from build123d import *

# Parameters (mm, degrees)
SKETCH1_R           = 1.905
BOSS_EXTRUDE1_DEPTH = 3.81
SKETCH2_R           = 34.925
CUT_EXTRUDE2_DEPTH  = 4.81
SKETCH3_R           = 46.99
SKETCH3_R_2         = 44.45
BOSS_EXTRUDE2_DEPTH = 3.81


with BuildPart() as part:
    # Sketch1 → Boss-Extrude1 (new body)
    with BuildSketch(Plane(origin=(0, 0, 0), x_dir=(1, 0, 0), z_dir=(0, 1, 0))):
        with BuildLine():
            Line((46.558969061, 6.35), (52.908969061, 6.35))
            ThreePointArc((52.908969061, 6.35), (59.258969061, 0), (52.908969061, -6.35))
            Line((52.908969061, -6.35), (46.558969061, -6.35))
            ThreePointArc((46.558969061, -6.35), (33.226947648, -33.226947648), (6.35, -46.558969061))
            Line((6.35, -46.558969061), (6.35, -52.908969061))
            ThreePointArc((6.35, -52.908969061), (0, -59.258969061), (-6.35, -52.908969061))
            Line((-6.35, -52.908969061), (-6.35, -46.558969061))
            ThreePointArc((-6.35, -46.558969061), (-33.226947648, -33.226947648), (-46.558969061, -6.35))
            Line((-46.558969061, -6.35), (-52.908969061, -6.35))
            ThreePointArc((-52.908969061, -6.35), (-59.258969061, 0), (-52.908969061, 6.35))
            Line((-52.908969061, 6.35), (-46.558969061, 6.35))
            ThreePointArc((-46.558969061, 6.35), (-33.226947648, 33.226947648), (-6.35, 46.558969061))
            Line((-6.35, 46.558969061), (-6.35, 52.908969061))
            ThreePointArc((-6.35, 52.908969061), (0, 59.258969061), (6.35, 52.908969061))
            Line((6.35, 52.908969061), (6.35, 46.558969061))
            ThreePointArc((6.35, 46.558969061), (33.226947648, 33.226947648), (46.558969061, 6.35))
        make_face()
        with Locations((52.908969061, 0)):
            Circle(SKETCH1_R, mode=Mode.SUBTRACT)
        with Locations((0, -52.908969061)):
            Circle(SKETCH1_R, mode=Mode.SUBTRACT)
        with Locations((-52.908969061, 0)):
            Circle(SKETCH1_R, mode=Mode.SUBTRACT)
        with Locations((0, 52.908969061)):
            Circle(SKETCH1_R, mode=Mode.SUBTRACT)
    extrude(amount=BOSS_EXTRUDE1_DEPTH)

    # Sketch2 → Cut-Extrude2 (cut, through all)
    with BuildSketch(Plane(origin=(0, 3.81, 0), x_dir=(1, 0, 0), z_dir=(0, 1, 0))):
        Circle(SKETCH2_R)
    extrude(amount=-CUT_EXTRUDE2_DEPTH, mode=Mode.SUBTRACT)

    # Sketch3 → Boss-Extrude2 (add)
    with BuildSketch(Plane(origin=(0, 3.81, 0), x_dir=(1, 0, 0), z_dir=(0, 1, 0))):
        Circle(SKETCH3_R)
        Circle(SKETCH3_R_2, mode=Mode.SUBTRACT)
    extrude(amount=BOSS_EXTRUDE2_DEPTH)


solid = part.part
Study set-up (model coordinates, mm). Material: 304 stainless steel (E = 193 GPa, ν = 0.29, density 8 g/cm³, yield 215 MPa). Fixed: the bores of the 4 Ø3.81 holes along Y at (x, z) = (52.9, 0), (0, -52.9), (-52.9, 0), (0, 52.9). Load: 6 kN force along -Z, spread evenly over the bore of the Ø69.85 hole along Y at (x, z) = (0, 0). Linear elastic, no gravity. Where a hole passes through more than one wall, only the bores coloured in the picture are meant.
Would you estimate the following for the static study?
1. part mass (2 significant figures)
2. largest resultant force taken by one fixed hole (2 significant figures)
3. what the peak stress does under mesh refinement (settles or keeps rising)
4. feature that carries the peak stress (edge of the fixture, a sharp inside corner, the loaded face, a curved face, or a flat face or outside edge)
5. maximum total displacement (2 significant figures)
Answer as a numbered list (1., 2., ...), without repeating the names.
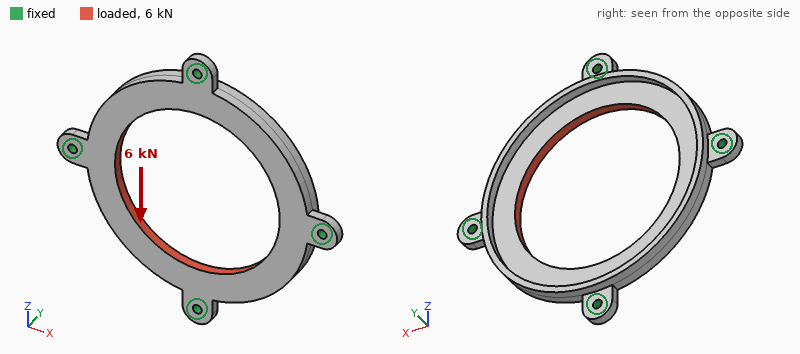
1. 130 g
2. 1.7 kN
3. keeps rising
4. edge of the fixture
5. 16 µm
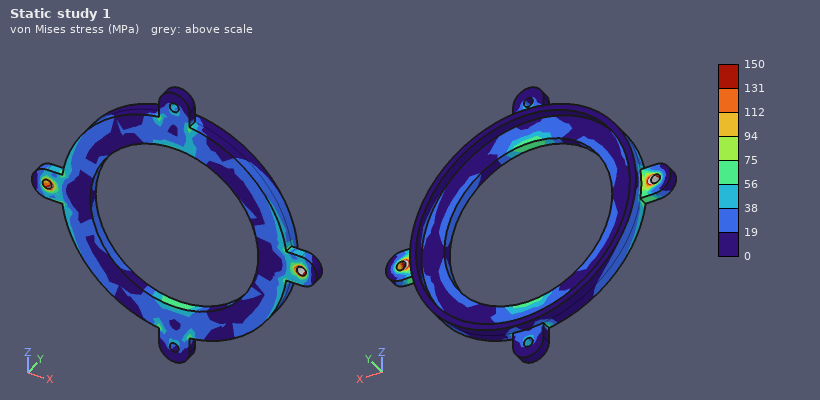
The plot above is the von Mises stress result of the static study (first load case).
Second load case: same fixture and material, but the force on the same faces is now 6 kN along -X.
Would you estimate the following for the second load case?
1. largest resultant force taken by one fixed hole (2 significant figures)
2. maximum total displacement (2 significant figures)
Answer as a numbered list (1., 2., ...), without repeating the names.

1. 1.7 kN
2. 16 µm
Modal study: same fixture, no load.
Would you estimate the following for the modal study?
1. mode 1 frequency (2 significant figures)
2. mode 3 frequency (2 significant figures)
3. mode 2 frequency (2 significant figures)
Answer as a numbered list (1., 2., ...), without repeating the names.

1. 3500 Hz
2. 4100 Hz
3. 4100 Hz
